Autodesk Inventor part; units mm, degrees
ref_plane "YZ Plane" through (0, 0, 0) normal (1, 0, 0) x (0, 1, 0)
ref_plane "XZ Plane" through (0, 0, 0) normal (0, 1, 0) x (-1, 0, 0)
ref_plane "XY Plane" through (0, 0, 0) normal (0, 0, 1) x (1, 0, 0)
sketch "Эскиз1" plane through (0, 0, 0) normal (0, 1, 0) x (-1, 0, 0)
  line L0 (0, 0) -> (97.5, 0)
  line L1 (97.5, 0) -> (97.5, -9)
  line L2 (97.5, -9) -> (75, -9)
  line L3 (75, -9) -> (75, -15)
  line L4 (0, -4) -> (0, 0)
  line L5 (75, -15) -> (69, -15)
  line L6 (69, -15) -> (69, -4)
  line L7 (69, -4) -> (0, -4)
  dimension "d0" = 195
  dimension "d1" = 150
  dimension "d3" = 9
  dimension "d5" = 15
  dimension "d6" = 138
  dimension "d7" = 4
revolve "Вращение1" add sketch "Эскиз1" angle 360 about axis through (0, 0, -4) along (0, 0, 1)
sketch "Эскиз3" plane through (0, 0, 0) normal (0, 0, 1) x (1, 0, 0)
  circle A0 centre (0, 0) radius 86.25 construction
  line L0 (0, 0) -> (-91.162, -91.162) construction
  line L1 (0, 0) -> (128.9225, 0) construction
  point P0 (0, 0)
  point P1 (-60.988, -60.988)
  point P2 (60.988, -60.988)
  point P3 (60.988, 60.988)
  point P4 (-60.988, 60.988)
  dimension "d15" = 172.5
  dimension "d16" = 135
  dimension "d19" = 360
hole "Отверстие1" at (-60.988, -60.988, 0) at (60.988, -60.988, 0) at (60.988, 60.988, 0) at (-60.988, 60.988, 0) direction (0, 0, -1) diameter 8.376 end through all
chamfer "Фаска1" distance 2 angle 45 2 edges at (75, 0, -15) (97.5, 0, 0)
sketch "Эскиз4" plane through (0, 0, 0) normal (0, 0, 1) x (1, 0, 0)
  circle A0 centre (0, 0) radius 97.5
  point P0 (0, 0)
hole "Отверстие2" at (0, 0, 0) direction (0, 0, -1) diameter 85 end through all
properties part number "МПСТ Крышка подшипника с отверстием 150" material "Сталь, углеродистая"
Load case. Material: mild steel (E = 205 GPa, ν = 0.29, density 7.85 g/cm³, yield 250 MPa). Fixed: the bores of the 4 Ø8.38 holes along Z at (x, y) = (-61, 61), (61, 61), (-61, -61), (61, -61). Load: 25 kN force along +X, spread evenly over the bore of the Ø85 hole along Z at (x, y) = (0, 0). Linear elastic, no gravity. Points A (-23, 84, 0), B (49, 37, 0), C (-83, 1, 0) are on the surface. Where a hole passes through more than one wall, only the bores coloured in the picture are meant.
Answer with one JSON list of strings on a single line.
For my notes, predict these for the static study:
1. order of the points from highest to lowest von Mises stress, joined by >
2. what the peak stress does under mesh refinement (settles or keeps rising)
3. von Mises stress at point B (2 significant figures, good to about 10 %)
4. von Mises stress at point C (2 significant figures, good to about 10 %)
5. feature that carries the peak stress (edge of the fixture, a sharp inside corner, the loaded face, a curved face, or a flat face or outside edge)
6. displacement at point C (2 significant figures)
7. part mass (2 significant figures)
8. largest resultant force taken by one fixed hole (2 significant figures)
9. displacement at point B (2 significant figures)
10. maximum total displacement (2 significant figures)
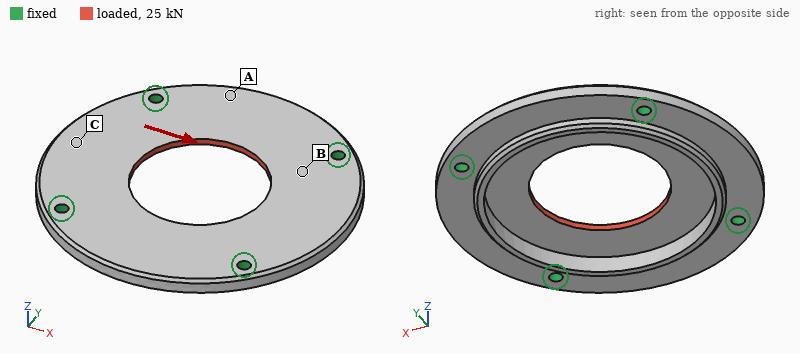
["B > C > A", "keeps rising", "27 MPa", "15 MPa", "edge of the fixture", "11 µm", "1.4 kg", "6.3 kN", "8.0 µm", "19 µm"]
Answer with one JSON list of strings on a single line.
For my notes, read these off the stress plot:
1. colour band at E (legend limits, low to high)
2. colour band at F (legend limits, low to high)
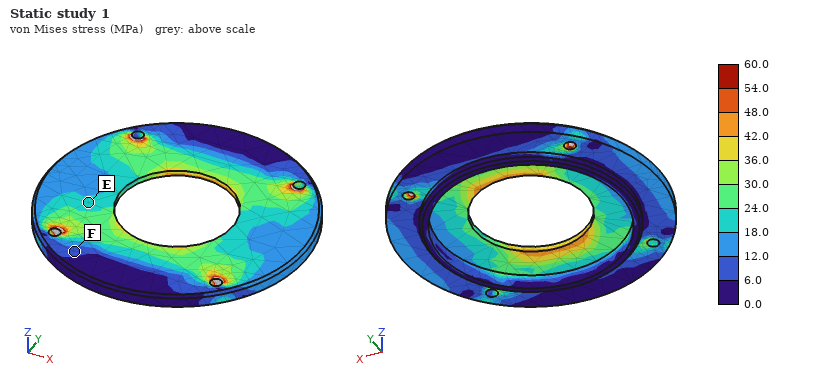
["18.0 to 24.0 MPa", "6.0 to 12.0 MPa"]
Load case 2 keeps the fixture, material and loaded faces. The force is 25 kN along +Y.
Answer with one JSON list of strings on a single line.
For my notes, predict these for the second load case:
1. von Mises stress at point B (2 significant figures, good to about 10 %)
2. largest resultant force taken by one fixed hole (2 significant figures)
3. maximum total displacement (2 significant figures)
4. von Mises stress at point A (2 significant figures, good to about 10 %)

["29 MPa", "6.3 kN", "19 µm", "16 MPa"]
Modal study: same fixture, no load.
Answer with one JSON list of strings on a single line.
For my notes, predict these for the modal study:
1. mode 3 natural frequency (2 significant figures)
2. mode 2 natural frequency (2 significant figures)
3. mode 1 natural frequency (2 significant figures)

["2900 Hz", "2900 Hz", "2600 Hz"]
